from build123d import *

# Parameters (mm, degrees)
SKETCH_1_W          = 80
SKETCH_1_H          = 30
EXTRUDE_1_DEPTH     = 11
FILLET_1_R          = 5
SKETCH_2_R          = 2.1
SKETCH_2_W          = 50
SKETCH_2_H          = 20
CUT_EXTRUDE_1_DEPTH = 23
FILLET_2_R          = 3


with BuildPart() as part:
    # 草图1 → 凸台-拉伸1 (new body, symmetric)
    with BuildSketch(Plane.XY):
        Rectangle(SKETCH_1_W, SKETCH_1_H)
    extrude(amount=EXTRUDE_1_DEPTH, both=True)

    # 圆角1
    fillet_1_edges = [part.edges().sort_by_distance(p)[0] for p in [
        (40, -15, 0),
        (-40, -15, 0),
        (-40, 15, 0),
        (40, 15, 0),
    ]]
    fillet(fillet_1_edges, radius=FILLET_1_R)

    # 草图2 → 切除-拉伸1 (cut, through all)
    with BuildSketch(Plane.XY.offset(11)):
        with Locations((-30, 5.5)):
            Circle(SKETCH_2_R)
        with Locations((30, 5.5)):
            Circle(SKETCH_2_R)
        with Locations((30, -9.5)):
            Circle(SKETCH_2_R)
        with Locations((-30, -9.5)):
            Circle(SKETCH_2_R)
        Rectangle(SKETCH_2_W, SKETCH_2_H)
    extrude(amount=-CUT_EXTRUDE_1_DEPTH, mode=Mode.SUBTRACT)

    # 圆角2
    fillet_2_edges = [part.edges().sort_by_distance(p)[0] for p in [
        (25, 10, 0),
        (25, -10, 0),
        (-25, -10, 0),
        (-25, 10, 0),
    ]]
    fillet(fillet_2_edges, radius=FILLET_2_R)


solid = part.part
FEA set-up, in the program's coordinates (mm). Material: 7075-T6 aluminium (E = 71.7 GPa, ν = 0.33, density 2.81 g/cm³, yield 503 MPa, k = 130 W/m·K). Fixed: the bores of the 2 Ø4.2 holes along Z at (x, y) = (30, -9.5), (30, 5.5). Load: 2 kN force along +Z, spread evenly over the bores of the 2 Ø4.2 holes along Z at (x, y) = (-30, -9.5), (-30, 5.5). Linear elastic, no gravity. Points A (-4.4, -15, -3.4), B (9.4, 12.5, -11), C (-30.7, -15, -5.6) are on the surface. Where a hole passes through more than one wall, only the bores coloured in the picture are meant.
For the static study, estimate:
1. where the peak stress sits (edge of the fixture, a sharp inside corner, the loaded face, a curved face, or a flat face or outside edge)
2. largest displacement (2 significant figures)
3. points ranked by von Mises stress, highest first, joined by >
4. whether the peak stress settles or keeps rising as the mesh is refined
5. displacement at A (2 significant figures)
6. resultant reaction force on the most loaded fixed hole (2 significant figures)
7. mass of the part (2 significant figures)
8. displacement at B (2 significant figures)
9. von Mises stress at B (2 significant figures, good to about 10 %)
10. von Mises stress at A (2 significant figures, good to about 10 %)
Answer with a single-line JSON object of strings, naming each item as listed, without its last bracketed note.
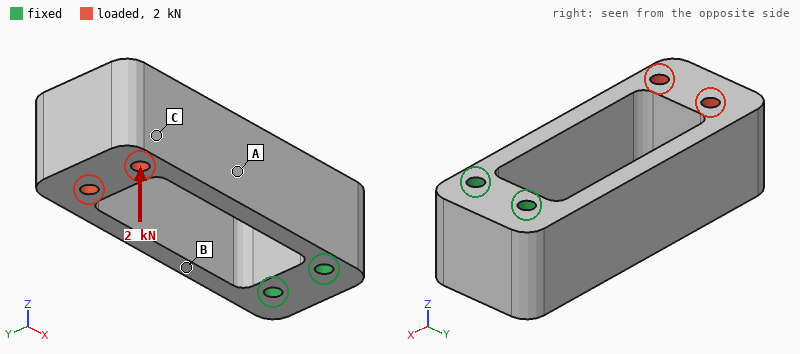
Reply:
{"where the peak stress sits": "edge of the fixture", "largest displacement": "0.33 mm", "points ranked by von Mises stress, highest first, joined by >": "B > A > C", "whether the peak stress settles or keeps rising as the mesh is refined": "keeps rising", "displacement at A": "0.11 mm", "resultant reaction force on the most loaded fixed hole": "1.0 kN", "mass of the part": "82 g", "displacement at B": "0.063 mm", "von Mises stress at B": "89 MPa", "von Mises stress at A": "38 MPa"}
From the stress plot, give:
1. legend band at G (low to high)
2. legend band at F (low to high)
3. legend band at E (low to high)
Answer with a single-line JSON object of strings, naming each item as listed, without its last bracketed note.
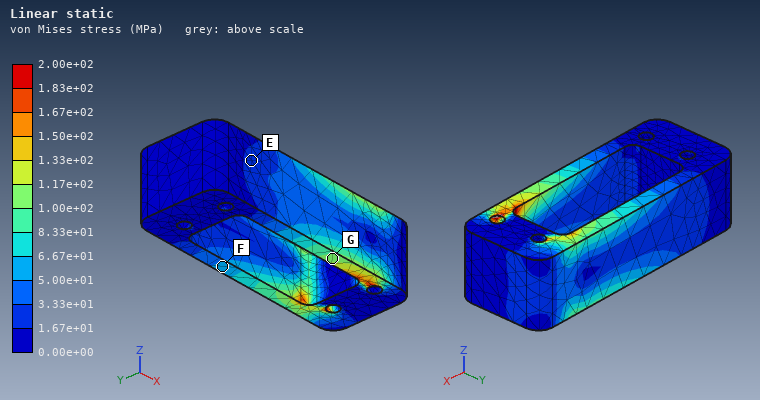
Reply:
{"legend band at G": "1.00e+02 to 1.17e+02 MPa", "legend band at F": "5.00e+01 to 6.67e+01 MPa", "legend band at E": "1.67e+01 to 3.33e+01 MPa"}
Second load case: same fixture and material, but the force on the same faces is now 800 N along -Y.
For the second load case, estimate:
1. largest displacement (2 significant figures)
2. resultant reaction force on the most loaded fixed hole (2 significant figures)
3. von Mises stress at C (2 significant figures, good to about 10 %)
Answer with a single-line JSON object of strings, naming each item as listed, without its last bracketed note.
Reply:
{"largest displacement": "0.33 mm", "resultant reaction force on the most loaded fixed hole": "2.2 kN", "von Mises stress at C": "20 MPa"}
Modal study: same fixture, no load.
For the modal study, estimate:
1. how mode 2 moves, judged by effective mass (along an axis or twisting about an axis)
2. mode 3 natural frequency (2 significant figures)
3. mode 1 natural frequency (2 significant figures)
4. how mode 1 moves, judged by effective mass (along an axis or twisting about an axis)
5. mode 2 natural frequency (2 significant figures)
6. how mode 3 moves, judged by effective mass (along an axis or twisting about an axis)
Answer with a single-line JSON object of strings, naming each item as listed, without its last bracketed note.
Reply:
{"how mode 2 moves, judged by effective mass": "along Z", "mode 3 natural frequency": "4700 Hz", "mode 1 natural frequency": "1300 Hz", "how mode 1 moves, judged by effective mass": "along Y", "mode 2 natural frequency": "2300 Hz", "how mode 3 moves, judged by effective mass": "twisting about X"}
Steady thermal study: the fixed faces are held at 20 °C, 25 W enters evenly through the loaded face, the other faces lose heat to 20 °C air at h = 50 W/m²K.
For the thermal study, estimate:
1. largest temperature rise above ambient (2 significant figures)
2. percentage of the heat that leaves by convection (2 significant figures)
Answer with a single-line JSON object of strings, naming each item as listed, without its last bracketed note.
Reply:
{"largest temperature rise above ambient": "37 K", "percentage of the heat that leaves by convection": "35 %"}
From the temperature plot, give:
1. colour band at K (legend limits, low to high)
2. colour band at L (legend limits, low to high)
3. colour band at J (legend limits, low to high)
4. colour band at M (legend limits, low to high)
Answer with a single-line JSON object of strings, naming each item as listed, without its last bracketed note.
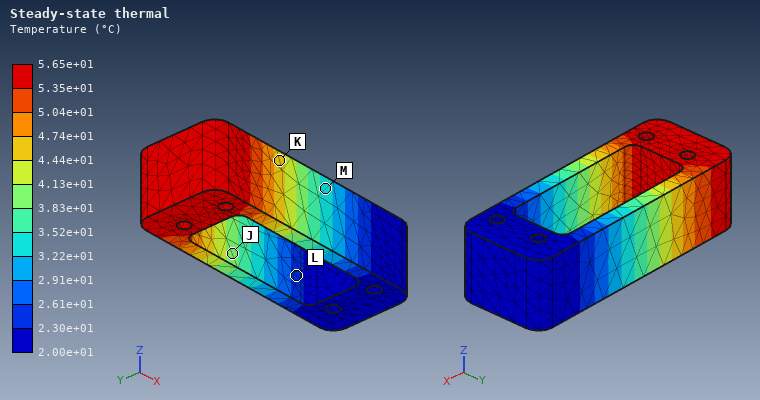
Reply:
{"colour band at K": "4.44e+01 to 4.74e+01 °C", "colour band at L": "2.30e+01 to 2.61e+01 °C", "colour band at J": "3.83e+01 to 4.13e+01 °C", "colour band at M": "3.22e+01 to 3.52e+01 °C"}
